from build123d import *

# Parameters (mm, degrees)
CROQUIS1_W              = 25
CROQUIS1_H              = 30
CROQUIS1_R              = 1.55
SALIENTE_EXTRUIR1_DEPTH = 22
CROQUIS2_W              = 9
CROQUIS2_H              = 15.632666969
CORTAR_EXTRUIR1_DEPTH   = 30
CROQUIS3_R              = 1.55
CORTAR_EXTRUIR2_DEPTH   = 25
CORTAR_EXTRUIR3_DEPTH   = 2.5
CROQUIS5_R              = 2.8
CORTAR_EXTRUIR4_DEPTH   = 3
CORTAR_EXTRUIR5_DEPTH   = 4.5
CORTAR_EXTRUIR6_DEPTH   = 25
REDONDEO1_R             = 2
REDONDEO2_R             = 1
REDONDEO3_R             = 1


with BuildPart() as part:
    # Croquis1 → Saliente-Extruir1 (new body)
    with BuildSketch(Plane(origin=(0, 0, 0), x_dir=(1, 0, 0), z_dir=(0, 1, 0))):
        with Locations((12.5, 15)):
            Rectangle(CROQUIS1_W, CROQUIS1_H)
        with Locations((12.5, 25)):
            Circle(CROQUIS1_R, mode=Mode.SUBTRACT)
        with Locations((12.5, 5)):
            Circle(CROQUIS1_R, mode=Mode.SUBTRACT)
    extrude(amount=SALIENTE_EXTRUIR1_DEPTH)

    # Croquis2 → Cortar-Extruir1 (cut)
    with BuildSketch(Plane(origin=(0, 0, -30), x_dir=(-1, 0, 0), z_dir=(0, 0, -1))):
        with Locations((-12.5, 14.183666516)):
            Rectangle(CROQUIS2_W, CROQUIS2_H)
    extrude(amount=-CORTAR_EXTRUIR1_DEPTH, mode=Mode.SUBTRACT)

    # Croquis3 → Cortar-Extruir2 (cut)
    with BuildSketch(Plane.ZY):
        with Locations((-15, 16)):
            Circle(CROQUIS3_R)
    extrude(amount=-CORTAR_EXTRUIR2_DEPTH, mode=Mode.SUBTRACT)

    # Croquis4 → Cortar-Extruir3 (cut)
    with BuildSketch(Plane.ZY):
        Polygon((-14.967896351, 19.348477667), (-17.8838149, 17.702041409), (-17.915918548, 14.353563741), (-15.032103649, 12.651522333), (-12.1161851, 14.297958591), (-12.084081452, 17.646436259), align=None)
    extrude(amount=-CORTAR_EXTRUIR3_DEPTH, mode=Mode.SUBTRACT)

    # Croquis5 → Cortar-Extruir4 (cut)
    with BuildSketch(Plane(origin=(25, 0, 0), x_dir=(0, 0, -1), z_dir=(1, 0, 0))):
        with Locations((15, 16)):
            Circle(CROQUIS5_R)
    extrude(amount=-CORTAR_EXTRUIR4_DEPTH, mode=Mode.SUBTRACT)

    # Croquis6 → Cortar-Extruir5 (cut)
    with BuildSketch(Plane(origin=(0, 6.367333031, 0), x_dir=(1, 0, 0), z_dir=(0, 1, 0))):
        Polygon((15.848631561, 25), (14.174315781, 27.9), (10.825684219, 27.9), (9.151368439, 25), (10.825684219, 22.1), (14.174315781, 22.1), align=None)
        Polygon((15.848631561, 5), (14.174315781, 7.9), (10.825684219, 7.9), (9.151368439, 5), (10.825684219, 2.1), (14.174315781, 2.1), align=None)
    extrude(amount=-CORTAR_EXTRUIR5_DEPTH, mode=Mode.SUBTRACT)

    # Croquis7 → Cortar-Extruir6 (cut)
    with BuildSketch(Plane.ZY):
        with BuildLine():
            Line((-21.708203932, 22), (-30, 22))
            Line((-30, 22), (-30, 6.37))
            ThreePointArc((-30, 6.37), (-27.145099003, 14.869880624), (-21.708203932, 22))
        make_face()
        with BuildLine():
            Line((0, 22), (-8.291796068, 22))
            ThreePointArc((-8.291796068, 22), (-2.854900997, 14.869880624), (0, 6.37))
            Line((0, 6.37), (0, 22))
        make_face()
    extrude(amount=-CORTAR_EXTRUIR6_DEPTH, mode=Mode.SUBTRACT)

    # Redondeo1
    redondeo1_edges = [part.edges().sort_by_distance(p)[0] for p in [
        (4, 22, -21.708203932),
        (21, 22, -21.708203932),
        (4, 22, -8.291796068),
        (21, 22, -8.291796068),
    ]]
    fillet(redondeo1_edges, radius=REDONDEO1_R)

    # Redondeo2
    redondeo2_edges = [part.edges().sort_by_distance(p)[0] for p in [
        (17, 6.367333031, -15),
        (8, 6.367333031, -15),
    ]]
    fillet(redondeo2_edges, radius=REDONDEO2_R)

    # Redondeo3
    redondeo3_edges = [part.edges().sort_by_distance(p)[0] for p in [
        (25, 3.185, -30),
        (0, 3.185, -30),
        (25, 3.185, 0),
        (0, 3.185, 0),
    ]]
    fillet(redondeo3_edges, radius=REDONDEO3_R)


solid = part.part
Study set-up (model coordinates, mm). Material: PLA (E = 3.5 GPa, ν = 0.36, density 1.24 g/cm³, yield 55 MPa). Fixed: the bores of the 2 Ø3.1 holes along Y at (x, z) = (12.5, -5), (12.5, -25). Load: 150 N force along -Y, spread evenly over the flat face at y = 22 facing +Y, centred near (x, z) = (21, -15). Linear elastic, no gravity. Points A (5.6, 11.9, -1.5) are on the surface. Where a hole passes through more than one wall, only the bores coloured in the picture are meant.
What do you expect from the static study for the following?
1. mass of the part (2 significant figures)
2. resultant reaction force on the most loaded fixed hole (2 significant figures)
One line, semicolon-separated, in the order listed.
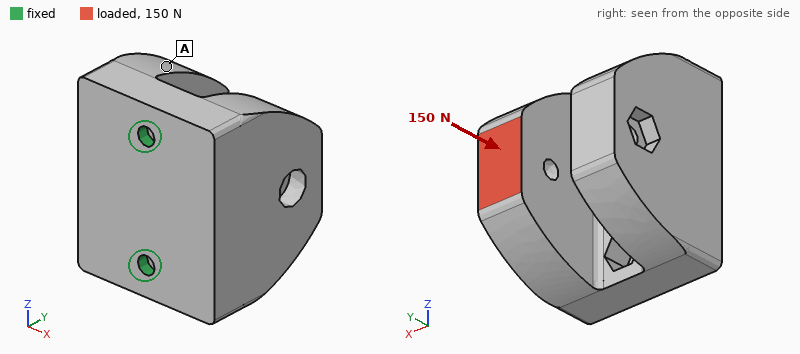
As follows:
13 g; 77 N
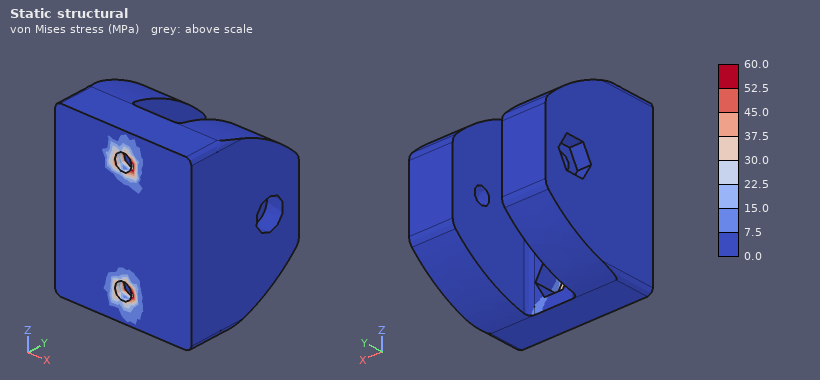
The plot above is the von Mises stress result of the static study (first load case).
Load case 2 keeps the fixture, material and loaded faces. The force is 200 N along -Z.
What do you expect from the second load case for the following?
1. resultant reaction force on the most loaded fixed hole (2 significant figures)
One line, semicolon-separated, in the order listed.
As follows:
240 N
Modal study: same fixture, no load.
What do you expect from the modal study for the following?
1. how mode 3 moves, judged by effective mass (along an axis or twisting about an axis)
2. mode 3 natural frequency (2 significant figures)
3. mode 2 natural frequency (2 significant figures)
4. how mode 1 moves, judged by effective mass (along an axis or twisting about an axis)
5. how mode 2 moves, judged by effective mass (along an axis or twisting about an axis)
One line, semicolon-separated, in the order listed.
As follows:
along Z; 4000 Hz; 3200 Hz; along X; along Y
